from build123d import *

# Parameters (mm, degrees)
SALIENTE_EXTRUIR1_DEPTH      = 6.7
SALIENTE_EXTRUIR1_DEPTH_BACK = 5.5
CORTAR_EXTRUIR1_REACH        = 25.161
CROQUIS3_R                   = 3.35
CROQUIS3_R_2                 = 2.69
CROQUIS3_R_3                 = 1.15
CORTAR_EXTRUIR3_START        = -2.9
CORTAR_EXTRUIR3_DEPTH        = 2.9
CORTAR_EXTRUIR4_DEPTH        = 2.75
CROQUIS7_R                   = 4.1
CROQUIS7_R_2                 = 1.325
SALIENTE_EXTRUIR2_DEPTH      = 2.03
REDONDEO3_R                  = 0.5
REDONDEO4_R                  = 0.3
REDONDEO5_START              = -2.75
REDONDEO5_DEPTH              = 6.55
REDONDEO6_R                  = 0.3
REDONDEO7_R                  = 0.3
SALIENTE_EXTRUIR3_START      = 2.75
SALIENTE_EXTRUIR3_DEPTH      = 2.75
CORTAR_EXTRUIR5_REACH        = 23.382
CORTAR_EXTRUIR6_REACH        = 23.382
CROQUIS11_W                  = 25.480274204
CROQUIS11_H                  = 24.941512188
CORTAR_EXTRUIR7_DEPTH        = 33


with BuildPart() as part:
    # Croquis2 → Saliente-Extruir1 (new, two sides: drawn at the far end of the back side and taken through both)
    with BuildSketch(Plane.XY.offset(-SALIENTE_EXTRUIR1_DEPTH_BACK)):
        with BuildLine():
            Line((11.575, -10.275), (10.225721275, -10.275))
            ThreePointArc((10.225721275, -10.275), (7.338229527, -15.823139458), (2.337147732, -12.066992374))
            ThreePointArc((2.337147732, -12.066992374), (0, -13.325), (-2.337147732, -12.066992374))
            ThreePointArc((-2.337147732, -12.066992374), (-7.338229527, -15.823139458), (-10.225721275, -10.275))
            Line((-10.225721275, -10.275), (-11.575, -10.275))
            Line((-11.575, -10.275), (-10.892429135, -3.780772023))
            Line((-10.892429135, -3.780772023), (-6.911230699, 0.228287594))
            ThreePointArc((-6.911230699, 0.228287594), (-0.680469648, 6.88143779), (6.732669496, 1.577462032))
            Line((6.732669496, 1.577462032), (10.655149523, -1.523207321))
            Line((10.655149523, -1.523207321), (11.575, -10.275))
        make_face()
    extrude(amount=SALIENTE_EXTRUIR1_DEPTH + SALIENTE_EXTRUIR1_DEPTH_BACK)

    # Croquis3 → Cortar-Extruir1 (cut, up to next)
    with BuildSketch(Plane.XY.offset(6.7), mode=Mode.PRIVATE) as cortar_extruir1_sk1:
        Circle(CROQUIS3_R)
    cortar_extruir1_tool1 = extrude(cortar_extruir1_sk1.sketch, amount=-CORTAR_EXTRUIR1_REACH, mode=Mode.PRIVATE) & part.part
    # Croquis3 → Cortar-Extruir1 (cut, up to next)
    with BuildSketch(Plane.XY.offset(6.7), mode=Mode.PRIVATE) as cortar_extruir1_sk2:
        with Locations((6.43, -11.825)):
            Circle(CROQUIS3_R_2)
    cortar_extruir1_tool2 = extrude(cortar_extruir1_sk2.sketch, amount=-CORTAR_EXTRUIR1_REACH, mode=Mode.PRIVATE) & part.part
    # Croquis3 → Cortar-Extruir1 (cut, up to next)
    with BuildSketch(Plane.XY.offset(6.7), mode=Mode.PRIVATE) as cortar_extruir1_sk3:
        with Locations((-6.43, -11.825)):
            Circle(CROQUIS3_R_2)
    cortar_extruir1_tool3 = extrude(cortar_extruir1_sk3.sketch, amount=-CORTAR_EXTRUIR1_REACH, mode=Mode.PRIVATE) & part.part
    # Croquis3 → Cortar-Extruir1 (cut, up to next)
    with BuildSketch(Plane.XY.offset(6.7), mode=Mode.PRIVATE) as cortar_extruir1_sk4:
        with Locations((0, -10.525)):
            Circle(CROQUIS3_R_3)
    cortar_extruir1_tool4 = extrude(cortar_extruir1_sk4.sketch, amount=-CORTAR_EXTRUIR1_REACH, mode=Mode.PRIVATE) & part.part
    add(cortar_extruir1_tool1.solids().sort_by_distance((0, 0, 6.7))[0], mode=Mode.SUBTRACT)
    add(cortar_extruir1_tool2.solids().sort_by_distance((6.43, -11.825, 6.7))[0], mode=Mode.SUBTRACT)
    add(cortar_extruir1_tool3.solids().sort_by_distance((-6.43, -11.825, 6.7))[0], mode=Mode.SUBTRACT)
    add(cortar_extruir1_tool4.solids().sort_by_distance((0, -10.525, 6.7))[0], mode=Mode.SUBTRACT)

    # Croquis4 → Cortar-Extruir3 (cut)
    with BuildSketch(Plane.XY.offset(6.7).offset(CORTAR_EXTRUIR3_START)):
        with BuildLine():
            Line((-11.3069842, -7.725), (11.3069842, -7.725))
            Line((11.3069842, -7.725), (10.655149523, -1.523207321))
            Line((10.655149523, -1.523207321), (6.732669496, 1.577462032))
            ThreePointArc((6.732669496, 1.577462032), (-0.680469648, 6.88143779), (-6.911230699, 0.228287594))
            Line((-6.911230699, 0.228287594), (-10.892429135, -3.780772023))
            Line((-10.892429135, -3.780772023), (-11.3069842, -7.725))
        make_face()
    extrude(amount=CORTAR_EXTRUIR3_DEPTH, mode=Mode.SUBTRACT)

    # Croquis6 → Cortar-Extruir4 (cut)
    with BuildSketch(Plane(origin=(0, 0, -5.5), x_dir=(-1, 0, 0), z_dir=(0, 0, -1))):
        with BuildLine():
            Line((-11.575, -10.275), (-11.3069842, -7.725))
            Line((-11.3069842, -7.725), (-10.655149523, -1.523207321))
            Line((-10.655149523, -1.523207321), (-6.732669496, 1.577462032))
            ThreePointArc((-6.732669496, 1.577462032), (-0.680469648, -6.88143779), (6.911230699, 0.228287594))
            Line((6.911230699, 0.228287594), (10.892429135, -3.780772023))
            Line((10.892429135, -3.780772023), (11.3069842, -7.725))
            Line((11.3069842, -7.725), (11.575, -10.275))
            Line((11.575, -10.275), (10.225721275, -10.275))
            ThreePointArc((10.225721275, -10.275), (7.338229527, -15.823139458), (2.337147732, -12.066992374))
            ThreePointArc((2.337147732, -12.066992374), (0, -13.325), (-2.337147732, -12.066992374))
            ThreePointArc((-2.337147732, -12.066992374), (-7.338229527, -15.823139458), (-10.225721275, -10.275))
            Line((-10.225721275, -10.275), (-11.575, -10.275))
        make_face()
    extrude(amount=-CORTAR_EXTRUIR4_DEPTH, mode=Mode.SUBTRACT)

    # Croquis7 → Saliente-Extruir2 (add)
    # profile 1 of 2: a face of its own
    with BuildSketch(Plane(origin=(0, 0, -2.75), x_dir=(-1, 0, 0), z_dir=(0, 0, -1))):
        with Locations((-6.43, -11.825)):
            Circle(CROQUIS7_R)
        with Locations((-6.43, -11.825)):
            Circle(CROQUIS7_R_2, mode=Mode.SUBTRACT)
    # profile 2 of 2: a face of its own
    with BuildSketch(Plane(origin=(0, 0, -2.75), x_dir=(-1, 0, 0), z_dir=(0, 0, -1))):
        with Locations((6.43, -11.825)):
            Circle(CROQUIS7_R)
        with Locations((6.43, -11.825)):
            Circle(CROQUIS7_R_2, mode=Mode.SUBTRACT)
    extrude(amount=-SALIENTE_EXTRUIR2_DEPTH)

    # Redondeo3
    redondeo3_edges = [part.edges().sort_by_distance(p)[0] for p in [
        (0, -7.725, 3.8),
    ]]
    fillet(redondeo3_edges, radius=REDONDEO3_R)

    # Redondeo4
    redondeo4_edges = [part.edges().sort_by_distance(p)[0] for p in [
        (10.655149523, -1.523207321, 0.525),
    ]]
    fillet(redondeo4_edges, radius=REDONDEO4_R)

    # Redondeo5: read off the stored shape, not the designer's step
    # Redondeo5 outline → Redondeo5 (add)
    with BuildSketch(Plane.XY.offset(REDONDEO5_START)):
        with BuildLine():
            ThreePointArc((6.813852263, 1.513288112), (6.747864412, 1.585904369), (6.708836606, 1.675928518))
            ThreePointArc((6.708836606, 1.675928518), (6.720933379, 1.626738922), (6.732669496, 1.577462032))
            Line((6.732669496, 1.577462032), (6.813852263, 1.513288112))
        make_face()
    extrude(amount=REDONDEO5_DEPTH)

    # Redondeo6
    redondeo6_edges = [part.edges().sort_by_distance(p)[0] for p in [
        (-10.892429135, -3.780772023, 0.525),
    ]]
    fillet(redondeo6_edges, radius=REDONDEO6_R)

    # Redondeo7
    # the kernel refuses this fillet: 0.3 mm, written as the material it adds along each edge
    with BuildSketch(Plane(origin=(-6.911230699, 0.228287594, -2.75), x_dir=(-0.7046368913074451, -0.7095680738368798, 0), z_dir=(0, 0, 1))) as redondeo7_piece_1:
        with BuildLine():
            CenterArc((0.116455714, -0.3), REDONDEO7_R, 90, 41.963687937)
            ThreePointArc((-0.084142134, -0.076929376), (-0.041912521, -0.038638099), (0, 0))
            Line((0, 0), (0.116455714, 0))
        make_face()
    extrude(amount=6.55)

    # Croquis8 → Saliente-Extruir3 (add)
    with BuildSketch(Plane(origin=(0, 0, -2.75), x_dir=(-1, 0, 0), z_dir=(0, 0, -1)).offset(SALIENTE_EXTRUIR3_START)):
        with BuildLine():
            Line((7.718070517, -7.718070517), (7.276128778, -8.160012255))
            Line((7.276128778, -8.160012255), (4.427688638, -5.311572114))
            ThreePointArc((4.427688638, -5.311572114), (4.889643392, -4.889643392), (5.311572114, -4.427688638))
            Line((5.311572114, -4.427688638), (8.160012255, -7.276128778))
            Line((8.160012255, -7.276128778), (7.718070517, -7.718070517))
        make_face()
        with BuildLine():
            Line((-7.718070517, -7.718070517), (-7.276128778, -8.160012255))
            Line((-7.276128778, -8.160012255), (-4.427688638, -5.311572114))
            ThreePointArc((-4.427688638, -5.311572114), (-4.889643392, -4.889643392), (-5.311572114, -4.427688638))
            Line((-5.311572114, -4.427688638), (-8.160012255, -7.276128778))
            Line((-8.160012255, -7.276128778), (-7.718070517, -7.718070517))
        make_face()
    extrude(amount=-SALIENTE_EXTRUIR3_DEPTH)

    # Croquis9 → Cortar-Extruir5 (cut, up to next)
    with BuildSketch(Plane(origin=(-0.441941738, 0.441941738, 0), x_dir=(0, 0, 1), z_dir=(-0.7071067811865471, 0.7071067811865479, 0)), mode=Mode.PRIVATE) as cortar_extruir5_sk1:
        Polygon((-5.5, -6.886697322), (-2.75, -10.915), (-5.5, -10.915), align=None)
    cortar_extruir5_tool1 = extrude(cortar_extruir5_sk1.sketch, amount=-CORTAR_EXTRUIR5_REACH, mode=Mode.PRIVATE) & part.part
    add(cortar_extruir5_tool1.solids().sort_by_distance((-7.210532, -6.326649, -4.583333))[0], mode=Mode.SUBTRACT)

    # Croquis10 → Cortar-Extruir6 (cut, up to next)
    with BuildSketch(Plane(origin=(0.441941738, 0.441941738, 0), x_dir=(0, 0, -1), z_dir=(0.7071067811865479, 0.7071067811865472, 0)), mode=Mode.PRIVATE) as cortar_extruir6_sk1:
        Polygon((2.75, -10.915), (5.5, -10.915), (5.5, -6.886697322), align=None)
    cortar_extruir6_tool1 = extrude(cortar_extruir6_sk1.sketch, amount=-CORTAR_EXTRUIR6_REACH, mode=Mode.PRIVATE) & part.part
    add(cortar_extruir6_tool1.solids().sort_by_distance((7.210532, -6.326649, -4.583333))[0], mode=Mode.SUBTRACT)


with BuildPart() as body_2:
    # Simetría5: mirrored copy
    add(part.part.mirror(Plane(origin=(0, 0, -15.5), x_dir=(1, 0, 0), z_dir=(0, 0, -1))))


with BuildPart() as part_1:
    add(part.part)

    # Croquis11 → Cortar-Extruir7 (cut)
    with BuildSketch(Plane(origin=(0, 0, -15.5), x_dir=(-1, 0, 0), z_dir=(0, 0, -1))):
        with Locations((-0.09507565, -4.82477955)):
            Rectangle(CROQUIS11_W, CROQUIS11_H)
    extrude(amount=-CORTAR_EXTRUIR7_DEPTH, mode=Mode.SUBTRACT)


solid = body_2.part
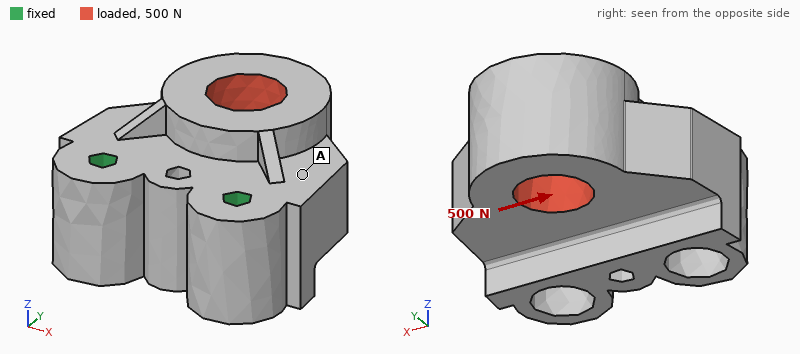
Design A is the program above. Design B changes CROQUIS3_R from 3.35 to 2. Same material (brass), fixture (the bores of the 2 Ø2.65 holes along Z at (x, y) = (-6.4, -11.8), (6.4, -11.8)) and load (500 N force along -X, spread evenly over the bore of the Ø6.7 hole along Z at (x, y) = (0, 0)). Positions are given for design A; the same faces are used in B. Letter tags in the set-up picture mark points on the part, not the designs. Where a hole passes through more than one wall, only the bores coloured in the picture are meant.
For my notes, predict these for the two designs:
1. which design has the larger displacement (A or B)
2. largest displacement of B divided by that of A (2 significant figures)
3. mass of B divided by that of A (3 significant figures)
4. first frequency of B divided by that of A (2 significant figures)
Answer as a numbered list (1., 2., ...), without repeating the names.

1. A
2. 0.87
3. 1.08
4. 0.95
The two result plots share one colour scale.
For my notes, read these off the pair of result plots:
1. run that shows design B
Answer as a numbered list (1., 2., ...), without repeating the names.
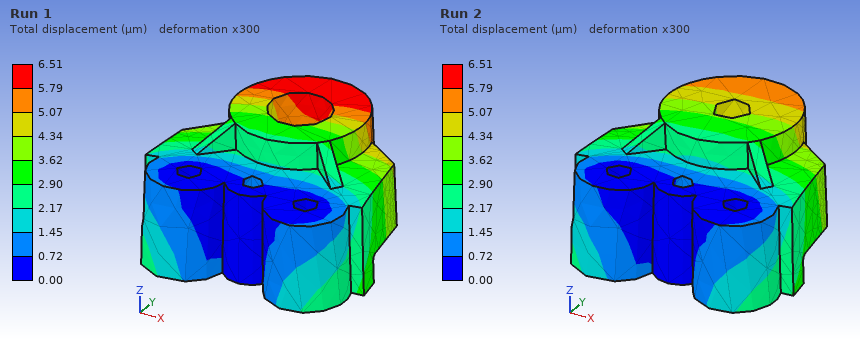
1. Run 2
